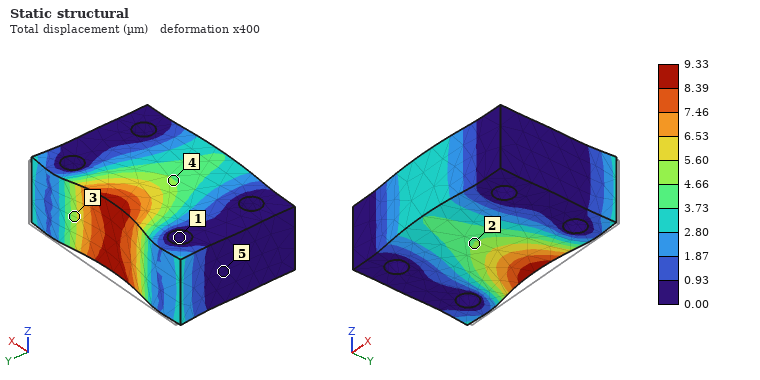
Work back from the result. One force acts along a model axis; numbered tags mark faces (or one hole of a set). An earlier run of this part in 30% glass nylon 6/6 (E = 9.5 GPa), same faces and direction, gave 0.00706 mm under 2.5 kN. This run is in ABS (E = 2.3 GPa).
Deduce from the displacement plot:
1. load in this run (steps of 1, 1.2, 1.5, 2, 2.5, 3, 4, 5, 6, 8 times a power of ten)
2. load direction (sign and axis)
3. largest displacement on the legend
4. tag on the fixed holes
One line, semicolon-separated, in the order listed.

800 N; -Y; 9.33 µm; 1
